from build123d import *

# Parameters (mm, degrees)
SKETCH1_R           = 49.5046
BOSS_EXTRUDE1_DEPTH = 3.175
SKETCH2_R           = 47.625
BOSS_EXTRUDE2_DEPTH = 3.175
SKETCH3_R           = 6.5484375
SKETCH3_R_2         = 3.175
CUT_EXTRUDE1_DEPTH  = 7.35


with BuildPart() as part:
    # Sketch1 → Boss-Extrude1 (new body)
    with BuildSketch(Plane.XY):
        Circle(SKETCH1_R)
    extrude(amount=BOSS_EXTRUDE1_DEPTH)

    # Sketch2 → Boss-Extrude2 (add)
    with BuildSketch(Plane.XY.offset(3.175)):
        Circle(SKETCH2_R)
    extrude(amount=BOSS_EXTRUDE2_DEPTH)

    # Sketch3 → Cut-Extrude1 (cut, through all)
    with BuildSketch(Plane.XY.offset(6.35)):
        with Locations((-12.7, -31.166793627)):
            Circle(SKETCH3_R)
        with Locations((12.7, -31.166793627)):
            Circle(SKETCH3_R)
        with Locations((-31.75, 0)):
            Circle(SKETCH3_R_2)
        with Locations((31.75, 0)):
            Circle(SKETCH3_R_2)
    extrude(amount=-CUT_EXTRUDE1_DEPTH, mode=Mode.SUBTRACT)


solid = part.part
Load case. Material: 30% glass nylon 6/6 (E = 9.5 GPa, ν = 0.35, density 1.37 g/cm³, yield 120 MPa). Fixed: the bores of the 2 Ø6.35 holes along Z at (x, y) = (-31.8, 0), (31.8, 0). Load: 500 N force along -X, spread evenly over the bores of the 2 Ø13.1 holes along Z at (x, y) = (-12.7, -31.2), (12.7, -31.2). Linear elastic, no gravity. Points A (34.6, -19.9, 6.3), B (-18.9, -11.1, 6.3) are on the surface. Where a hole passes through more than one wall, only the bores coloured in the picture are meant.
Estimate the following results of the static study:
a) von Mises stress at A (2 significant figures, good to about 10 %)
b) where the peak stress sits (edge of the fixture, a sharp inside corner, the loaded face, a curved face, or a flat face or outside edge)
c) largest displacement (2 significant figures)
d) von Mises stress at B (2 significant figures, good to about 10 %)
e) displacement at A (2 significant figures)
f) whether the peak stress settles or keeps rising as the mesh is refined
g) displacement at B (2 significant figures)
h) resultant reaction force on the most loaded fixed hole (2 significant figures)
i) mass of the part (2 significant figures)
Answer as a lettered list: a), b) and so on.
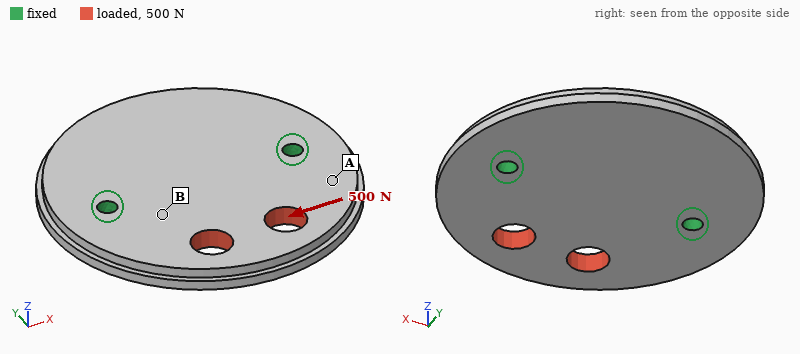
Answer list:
a) 1.1 MPa
b) edge of the fixture
c) 17 µm
d) 2.1 MPa
e) 7.9 µm
f) keeps rising
g) 4.5 µm
h) 340 N
i) 62 g
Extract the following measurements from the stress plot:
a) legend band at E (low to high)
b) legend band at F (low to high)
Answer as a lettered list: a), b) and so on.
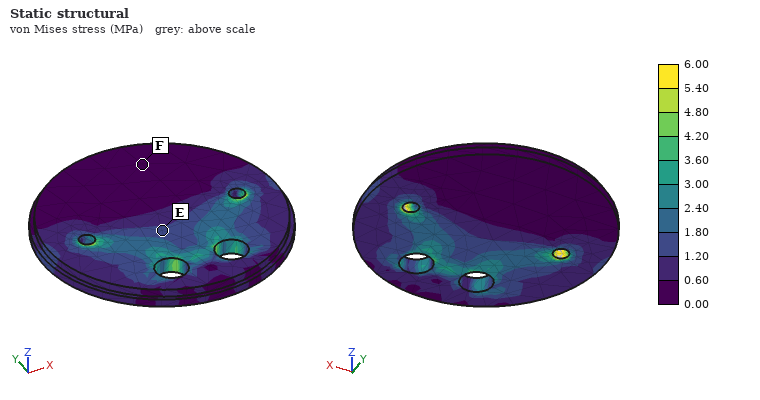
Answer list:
a) 1.20 to 1.80 MPa
b) 0.00 to 0.60 MPa
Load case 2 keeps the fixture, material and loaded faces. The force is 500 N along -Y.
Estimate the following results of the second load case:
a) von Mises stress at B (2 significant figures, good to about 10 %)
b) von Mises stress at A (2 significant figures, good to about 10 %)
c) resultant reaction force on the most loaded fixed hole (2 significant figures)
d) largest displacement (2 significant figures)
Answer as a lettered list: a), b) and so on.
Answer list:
a) 1.3 MPa
b) 0.71 MPa
c) 260 N
d) 8.8 µm
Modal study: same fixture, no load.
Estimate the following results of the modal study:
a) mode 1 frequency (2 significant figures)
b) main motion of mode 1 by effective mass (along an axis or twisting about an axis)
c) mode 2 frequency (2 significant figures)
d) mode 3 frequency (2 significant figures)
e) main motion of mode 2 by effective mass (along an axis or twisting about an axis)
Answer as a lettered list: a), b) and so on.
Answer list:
a) 1200 Hz
b) twisting about X
c) 1500 Hz
d) 2800 Hz
e) along Z
